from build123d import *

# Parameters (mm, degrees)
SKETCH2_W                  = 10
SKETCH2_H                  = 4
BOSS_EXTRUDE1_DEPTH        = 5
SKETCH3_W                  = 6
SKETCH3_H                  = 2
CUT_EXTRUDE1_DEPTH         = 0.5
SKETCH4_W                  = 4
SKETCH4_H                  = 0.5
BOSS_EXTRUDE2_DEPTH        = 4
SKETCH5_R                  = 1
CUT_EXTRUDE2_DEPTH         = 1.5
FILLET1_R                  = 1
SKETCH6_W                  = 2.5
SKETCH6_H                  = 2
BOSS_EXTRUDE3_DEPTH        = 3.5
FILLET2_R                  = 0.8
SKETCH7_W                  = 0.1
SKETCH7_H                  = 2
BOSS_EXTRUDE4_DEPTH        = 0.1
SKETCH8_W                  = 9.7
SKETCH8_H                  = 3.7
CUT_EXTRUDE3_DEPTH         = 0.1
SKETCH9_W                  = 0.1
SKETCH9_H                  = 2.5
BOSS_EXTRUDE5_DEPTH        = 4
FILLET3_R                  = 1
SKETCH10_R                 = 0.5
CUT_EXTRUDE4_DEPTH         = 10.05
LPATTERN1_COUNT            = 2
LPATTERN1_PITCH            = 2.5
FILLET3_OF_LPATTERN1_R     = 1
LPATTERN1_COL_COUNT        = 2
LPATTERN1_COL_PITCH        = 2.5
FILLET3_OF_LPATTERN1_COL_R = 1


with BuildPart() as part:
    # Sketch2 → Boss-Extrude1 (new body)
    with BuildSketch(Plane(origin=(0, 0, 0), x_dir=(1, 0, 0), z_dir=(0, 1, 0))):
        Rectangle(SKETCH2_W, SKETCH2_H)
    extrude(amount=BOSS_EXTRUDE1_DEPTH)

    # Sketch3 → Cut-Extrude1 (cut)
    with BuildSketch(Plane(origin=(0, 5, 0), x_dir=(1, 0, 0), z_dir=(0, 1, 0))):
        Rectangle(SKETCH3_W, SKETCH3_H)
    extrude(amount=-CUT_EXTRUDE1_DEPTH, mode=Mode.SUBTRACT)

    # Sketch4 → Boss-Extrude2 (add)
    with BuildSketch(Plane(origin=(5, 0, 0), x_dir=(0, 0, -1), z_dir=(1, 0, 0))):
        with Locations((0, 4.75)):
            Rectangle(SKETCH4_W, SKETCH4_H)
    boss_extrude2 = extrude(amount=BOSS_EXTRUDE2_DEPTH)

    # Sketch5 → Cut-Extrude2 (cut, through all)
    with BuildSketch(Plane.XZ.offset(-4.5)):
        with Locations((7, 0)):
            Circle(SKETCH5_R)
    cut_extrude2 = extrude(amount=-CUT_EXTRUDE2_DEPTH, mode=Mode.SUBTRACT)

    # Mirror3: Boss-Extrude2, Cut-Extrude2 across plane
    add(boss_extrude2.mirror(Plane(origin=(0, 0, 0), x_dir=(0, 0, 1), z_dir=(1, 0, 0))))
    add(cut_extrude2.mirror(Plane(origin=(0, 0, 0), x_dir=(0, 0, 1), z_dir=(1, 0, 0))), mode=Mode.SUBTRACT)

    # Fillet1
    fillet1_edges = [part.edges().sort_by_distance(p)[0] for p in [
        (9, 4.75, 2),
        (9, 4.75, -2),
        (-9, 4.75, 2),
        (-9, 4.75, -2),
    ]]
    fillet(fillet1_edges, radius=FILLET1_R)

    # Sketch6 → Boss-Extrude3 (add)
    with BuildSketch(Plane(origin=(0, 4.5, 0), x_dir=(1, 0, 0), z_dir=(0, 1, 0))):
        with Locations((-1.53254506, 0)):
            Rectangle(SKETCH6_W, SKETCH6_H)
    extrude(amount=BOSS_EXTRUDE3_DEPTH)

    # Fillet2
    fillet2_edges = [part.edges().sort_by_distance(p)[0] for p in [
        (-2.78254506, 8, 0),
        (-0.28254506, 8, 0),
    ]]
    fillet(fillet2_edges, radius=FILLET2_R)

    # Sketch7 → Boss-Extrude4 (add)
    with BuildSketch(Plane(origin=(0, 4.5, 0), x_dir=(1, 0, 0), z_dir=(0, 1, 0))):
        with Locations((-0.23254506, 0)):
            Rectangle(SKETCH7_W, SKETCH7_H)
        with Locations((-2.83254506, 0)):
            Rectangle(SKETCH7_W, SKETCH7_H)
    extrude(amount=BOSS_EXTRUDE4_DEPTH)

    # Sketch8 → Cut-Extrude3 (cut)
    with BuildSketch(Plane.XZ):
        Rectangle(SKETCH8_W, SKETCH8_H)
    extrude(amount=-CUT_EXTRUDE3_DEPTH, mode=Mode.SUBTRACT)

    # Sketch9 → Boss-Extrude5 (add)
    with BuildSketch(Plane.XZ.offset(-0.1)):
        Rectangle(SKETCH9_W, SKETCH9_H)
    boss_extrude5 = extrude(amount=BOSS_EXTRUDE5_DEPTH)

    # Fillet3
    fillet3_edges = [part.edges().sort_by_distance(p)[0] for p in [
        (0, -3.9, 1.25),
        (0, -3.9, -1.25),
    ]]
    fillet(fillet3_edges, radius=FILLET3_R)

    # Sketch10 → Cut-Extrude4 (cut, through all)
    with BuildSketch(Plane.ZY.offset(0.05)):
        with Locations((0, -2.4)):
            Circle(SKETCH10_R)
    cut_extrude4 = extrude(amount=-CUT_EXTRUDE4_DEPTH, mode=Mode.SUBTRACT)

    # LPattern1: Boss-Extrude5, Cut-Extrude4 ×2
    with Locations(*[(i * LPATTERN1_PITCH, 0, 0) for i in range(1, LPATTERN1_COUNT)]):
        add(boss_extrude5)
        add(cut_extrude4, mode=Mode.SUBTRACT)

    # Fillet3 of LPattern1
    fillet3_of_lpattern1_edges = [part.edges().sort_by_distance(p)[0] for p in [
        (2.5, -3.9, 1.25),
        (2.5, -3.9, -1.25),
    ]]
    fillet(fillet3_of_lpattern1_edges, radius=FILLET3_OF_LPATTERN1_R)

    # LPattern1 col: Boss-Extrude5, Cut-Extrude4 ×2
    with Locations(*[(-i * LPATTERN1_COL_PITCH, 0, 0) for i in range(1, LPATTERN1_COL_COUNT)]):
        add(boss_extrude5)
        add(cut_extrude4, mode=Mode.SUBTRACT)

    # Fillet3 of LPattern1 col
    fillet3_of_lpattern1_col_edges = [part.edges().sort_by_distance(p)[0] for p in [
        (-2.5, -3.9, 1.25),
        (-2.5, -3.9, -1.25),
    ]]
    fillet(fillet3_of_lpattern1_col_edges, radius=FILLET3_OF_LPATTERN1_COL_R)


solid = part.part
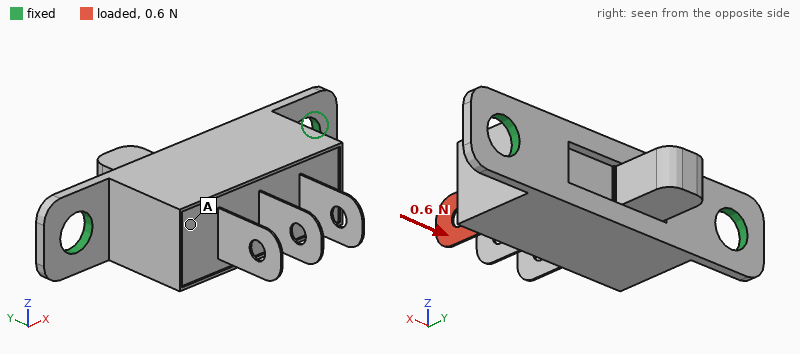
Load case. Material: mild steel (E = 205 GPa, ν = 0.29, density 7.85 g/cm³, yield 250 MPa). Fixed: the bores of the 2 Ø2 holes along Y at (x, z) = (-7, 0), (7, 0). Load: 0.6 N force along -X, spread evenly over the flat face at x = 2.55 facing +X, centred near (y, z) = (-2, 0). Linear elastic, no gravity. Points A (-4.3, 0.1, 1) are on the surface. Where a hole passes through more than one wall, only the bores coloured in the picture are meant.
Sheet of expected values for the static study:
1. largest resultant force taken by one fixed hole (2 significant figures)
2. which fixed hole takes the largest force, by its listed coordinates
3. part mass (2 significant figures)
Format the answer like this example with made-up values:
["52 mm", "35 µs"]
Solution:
["0.52 N", "(-7, 0)", "1.7 g"]
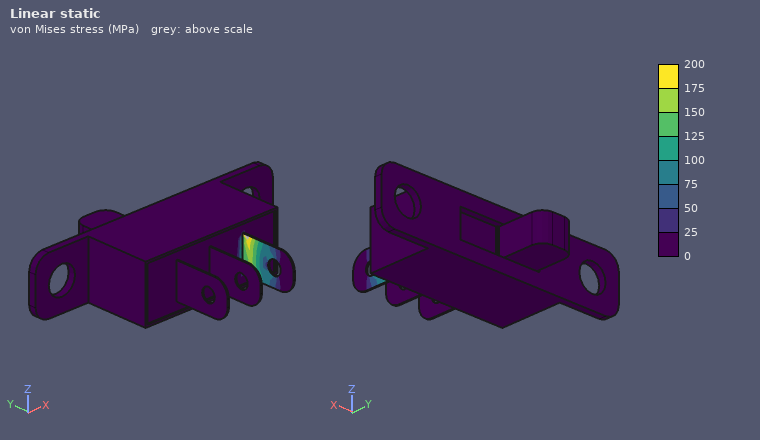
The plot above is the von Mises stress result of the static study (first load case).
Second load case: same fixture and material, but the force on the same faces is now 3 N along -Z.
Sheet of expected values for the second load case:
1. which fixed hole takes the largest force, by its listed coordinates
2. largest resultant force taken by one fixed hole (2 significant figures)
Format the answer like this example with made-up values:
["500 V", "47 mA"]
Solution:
["(7, 0)", "2.1 N"]
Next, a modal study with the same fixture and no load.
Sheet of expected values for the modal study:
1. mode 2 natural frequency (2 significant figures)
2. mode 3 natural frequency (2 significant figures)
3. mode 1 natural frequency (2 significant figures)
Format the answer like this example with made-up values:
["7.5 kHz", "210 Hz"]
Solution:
["5800 Hz", "5900 Hz", "5800 Hz"]
